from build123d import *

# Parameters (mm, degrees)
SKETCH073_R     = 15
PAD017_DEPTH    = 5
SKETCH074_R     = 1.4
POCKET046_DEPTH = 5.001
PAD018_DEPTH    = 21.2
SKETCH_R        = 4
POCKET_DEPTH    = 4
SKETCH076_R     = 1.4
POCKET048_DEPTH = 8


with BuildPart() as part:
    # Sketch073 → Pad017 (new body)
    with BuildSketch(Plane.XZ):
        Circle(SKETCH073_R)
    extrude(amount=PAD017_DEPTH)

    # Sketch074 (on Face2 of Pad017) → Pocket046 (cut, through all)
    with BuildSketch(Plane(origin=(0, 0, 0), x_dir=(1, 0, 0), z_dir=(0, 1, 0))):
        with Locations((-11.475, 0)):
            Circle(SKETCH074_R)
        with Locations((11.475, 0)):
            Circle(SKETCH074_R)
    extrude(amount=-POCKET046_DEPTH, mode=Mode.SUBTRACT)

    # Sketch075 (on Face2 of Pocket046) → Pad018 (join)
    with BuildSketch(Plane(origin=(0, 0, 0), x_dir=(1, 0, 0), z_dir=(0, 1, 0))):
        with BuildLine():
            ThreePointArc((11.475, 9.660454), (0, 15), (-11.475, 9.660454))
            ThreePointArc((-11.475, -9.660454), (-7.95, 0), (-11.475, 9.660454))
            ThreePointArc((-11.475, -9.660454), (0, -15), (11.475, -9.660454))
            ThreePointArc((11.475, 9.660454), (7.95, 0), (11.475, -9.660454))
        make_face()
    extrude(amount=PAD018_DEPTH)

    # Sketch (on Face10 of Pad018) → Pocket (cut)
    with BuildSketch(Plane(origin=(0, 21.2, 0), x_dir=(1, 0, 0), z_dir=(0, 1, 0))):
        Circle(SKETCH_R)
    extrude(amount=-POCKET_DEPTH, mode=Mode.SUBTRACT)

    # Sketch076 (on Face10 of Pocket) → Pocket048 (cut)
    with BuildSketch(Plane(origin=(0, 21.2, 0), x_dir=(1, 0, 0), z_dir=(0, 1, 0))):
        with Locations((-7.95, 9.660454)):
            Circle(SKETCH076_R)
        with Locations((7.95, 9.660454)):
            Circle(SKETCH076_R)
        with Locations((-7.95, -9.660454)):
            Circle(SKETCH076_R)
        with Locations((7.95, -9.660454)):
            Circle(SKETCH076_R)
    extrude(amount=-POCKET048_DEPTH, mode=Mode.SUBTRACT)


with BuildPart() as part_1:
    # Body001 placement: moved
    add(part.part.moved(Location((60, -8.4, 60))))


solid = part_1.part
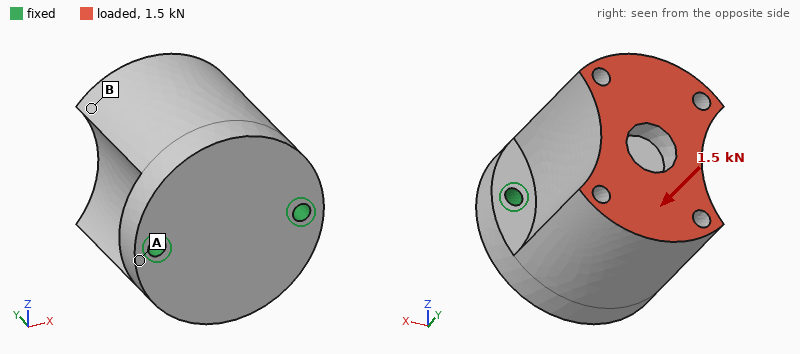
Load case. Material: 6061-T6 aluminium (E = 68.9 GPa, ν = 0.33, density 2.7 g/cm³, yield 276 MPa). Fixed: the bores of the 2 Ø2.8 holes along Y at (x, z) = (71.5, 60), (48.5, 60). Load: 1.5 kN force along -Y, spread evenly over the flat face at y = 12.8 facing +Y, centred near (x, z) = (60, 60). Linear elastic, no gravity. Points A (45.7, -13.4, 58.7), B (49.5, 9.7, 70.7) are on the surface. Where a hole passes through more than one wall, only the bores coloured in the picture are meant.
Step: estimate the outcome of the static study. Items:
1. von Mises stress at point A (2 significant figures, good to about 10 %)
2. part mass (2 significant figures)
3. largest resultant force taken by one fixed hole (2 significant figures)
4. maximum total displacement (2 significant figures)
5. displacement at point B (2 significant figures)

18 MPa
38 g
780 N
5.1 µm
4.9 µm
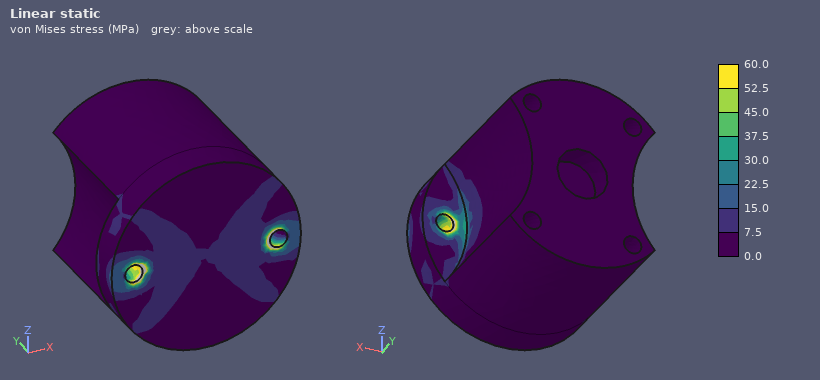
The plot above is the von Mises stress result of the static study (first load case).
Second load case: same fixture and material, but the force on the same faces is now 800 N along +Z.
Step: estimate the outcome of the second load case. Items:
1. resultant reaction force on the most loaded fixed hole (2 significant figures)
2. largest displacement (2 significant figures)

400 N
93 µm
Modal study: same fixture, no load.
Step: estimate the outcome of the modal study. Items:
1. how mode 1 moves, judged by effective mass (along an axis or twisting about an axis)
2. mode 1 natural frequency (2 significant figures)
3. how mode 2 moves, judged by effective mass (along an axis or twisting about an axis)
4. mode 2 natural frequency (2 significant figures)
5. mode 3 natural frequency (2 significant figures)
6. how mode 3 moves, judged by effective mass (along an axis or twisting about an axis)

along Z
4200 Hz
along X
11 kHz
16 kHz
along Y
